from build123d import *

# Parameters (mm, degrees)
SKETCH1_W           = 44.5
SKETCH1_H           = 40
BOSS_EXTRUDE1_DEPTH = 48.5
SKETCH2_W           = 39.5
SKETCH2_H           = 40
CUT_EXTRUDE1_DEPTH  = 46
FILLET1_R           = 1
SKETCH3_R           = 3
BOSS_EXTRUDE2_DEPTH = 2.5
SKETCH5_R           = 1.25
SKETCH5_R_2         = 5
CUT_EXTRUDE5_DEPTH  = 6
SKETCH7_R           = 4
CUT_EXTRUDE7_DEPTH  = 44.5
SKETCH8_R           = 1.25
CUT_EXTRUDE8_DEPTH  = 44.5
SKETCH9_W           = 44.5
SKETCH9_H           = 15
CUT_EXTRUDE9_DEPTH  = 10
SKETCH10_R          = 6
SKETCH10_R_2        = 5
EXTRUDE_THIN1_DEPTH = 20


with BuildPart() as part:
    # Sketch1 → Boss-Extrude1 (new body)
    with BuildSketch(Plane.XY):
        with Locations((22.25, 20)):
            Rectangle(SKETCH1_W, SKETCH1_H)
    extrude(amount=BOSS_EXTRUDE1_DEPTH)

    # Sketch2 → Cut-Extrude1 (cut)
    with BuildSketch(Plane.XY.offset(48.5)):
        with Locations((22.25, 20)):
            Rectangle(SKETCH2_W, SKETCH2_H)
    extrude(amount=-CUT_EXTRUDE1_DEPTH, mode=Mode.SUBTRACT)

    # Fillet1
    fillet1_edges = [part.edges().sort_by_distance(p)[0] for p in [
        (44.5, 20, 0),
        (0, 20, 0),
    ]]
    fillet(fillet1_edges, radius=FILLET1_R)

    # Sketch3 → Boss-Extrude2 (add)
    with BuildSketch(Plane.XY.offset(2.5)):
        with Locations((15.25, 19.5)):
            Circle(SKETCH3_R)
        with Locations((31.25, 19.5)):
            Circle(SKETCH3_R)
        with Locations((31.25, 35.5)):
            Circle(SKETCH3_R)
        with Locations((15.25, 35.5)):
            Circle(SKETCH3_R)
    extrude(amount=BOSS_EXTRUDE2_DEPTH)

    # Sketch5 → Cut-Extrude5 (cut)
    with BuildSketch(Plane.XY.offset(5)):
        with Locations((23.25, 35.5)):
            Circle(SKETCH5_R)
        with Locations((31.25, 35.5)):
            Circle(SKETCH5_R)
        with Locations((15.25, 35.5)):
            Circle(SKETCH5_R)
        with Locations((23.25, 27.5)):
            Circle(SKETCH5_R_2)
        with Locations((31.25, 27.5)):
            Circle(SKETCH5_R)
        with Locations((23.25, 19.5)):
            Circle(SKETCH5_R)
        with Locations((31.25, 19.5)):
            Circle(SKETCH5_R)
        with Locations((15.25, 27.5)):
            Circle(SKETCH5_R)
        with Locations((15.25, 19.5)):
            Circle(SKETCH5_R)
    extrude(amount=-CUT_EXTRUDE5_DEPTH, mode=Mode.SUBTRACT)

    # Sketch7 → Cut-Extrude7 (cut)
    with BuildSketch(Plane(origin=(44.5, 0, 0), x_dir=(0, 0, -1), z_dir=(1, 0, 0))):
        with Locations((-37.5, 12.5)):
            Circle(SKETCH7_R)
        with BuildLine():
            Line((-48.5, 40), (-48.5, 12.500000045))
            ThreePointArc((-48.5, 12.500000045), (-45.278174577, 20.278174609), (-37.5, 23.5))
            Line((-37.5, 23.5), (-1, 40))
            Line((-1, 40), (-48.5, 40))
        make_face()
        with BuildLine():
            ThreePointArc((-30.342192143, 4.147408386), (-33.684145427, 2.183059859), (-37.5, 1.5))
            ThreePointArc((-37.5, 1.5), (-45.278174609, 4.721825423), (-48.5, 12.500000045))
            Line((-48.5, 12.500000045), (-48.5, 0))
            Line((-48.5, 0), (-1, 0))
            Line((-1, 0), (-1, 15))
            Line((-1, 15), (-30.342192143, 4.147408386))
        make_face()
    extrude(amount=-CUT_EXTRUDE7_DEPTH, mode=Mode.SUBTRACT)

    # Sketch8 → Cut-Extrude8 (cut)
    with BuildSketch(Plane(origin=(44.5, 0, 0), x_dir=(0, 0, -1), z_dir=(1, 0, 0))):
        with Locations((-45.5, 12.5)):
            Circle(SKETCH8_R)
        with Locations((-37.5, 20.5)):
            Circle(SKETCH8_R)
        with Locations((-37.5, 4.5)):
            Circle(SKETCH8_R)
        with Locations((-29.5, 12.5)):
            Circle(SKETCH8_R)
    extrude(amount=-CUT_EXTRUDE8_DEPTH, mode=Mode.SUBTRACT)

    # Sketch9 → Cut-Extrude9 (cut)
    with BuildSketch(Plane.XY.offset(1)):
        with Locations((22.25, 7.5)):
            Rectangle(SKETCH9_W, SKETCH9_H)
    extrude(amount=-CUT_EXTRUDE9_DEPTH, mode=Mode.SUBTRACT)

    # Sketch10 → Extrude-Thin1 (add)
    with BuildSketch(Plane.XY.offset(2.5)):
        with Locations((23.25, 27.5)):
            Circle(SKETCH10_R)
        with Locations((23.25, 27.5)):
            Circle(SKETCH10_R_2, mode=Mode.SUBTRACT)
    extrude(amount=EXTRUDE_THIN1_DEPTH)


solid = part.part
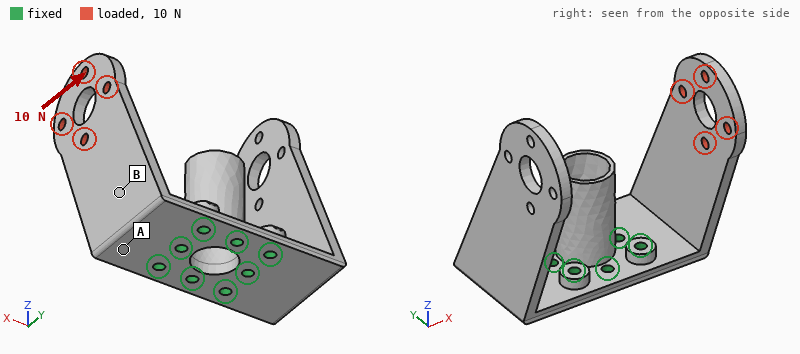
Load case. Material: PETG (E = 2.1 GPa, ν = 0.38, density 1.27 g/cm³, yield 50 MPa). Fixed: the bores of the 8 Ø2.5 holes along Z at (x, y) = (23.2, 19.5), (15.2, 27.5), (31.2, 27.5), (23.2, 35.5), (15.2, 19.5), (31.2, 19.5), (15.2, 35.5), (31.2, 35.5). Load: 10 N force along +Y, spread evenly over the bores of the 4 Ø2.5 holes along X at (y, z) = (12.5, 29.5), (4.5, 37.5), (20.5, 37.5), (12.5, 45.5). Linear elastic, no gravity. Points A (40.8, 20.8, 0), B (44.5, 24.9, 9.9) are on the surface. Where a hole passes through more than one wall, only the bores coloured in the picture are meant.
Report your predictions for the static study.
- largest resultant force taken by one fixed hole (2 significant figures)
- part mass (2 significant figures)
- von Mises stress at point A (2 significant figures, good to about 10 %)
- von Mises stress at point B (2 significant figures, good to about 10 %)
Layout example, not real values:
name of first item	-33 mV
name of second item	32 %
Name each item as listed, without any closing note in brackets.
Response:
largest resultant force taken by one fixed hole	23 N
part mass	10 g
von Mises stress at point A	5.1 MPa
von Mises stress at point B	0.86 MPa
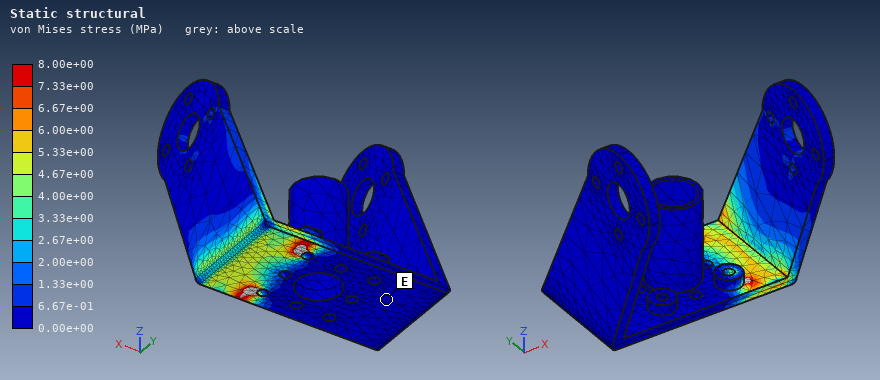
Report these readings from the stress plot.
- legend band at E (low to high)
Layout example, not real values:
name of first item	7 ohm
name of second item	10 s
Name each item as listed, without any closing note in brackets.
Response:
legend band at E	0.00e+00 to 6.67e-01 MPa
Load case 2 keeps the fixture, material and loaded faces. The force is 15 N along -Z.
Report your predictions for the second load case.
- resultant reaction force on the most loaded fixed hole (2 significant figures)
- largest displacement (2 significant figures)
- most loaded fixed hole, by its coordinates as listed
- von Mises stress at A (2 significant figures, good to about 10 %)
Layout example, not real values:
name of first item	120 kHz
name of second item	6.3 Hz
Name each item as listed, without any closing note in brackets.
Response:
resultant reaction force on the most loaded fixed hole	21 N
largest displacement	0.87 mm
most loaded fixed hole, by its coordinates as listed	(31.2, 19.5)
von Mises stress at A	3.5 MPa
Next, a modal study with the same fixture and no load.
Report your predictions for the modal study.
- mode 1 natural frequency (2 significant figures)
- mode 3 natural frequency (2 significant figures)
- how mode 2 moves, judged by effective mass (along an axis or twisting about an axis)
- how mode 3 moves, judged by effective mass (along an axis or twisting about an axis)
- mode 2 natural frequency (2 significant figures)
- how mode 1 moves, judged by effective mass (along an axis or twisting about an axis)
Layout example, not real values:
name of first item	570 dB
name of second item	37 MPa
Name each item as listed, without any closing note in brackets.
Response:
mode 1 natural frequency	190 Hz
mode 3 natural frequency	440 Hz
how mode 2 moves, judged by effective mass	along X
how mode 3 moves, judged by effective mass	along Y
mode 2 natural frequency	200 Hz
how mode 1 moves, judged by effective mass	along X
